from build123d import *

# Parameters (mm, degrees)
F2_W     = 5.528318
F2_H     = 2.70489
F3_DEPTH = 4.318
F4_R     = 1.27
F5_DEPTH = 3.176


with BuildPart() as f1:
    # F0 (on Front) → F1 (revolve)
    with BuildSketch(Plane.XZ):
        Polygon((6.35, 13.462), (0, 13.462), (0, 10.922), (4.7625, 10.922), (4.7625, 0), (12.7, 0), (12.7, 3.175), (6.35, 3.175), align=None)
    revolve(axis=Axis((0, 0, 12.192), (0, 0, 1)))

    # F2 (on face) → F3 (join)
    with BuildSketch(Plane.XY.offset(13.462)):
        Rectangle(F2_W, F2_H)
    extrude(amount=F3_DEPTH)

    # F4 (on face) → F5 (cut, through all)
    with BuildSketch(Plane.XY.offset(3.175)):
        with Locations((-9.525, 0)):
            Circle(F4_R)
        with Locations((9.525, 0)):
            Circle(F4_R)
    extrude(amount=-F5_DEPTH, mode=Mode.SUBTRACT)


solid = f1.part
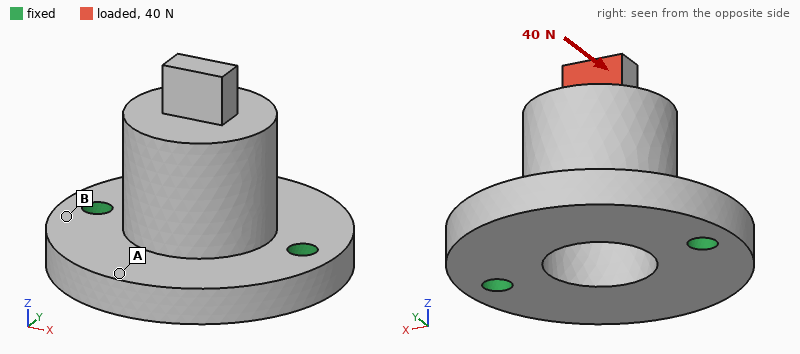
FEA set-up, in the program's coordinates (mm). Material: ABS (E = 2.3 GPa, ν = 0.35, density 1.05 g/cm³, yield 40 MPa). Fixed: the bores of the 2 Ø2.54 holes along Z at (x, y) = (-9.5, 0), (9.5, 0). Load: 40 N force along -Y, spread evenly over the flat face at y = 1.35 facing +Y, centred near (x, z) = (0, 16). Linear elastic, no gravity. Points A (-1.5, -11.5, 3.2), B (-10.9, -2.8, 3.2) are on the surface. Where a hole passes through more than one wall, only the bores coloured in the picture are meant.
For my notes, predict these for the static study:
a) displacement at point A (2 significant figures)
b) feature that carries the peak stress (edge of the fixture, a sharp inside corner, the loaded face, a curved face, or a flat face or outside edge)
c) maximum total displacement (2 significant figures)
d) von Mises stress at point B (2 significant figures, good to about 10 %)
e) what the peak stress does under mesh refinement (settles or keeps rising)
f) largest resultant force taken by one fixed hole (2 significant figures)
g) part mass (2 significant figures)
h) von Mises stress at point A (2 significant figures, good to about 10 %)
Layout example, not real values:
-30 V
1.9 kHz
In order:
0.13 mm
edge of the fixture
0.27 mm
6.6 MPa
keeps rising
20 N
2.3 g
2.4 MPa
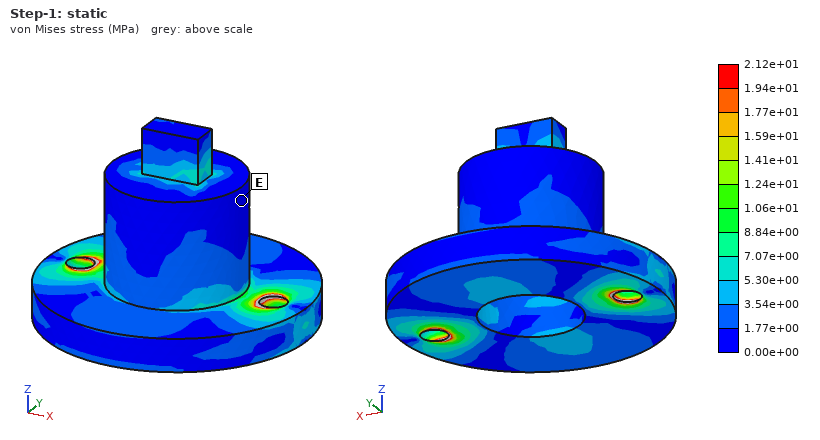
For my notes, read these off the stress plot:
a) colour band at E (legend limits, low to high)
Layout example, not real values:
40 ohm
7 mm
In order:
0.00e+00 to 1.77e+00 MPa
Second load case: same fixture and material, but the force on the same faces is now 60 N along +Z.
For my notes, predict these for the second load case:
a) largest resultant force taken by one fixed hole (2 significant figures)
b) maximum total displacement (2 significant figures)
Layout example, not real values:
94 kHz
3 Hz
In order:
31 N
88 µm
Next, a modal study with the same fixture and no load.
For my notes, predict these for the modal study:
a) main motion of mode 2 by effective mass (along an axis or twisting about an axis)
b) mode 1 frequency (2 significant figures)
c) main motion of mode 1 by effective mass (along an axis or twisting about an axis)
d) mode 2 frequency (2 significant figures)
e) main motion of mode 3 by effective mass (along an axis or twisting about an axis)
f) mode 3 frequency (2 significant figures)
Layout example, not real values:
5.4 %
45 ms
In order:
along Z
2900 Hz
along Y
6300 Hz
along X
6900 Hz
